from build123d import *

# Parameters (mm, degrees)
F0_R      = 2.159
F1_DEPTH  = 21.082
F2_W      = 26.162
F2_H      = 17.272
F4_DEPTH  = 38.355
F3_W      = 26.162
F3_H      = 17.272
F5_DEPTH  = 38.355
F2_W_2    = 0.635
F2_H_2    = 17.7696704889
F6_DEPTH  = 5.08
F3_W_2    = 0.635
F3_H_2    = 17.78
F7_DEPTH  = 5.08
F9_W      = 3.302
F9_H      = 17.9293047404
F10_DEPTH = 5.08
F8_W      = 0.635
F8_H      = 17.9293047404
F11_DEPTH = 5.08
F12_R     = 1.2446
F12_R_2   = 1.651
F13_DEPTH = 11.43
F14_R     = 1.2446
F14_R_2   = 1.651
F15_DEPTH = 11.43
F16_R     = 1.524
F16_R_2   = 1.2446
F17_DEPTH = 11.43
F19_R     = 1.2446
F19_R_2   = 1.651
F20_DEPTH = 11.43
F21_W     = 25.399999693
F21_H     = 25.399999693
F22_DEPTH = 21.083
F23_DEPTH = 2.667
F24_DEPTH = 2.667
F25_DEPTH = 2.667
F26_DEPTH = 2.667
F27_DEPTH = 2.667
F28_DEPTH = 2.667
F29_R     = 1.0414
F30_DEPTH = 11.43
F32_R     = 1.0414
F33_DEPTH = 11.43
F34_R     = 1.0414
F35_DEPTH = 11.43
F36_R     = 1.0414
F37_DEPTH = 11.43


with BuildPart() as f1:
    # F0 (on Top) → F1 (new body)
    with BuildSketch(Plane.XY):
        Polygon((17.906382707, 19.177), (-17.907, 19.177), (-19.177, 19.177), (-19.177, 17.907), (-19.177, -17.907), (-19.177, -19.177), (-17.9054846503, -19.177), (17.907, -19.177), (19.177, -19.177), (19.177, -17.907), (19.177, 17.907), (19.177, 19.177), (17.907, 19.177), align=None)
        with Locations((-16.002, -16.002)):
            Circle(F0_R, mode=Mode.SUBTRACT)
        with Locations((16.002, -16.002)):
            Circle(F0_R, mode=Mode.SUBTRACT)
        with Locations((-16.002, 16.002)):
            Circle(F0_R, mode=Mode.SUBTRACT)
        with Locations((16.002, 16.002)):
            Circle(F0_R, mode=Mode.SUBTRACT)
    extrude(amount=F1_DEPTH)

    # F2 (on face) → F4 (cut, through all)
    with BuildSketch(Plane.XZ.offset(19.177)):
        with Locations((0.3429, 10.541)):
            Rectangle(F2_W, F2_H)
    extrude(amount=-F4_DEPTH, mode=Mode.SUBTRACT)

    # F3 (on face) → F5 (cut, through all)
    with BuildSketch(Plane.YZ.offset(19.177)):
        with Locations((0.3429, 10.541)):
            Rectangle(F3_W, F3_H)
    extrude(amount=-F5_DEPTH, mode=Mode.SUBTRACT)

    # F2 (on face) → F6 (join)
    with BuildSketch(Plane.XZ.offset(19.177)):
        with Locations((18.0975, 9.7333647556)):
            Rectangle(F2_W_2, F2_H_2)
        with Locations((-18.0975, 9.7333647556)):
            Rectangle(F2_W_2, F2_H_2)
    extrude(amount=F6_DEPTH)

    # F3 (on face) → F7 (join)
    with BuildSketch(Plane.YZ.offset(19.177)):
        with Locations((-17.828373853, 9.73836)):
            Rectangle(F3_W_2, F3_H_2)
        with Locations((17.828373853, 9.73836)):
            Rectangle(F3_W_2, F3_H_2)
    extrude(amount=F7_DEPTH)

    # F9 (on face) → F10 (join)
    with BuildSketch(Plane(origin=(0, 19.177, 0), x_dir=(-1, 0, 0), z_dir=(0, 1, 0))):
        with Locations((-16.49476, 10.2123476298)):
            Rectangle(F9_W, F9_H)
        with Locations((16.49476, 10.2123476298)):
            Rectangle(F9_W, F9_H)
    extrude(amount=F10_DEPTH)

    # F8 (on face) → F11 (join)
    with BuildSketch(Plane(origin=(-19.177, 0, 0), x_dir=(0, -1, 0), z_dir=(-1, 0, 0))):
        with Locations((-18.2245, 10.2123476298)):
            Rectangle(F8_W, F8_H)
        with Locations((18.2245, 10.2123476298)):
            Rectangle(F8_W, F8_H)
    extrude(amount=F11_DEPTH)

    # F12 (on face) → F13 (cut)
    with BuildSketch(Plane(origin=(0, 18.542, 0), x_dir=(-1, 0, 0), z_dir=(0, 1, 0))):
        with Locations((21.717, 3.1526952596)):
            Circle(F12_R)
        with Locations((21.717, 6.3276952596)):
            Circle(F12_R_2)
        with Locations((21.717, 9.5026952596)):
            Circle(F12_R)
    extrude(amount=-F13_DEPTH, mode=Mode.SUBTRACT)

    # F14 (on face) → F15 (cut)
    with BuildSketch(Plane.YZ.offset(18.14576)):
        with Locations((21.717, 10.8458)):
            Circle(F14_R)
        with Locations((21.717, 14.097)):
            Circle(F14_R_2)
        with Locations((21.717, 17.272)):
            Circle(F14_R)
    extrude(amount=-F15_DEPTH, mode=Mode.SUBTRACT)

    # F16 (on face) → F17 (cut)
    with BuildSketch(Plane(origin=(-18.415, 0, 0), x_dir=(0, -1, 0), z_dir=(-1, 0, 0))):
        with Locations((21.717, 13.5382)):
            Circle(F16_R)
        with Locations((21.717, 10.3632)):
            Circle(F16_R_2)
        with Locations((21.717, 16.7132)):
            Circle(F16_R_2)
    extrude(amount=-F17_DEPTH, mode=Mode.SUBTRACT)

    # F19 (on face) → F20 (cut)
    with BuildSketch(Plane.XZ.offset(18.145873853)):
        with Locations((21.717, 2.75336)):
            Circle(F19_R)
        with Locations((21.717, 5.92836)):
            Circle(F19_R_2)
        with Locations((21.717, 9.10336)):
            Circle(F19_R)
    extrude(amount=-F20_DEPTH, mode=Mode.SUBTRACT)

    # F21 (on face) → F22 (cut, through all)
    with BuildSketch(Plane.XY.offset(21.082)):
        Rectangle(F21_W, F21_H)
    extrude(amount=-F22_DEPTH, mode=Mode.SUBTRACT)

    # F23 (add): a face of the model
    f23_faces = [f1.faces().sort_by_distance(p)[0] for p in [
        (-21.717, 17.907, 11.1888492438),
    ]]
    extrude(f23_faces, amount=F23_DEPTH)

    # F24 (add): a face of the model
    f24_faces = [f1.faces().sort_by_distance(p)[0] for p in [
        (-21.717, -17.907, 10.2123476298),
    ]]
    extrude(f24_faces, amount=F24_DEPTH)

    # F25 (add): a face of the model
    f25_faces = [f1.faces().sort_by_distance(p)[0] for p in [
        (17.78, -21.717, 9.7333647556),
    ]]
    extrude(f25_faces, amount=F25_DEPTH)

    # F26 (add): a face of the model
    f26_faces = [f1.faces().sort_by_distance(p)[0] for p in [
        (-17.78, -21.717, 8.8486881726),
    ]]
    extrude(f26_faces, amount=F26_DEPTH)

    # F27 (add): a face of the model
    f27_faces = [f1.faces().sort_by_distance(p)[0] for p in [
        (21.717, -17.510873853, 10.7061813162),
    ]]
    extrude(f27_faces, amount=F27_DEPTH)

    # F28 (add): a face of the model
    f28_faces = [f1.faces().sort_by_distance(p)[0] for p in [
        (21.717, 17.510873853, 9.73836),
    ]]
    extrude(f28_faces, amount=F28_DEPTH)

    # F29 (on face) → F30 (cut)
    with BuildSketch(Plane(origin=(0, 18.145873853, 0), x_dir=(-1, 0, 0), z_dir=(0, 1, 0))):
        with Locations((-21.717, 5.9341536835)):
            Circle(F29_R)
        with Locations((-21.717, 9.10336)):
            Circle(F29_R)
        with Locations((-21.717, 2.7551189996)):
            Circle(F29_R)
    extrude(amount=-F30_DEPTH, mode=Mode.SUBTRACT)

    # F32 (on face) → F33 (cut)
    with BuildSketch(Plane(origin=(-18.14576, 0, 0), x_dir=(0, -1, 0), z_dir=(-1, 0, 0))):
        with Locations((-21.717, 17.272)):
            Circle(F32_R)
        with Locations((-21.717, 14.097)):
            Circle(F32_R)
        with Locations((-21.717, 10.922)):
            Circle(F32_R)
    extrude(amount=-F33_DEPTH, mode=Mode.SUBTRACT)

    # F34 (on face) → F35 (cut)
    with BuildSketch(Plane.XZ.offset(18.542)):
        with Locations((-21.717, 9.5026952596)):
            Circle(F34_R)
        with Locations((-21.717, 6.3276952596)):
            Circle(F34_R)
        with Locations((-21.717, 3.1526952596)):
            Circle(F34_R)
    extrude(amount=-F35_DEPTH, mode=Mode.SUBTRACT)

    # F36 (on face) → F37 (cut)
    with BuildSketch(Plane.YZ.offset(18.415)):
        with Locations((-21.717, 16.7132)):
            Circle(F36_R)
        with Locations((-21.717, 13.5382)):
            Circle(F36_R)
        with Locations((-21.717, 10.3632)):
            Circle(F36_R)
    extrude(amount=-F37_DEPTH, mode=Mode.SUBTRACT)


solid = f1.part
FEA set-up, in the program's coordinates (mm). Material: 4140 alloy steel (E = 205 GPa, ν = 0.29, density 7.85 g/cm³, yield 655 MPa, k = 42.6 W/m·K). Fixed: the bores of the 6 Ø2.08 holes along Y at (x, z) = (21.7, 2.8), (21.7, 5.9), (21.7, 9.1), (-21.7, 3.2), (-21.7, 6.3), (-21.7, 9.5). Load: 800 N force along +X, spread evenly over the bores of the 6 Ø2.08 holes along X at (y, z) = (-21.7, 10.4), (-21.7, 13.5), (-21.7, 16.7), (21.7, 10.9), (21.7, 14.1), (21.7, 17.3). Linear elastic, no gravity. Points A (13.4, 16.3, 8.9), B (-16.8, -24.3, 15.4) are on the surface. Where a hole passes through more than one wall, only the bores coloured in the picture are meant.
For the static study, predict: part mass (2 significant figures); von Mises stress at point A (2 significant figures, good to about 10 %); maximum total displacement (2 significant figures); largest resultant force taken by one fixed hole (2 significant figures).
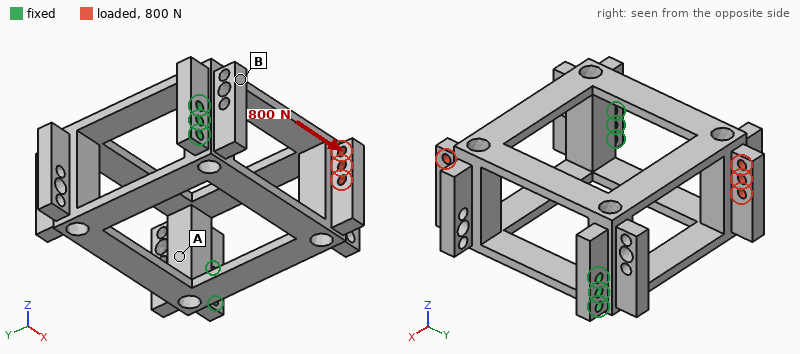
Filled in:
51 g
28 MPa
22 µm
550 N
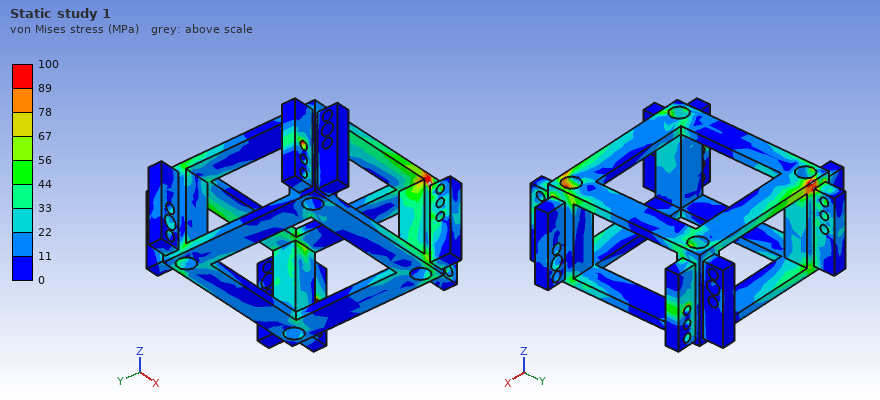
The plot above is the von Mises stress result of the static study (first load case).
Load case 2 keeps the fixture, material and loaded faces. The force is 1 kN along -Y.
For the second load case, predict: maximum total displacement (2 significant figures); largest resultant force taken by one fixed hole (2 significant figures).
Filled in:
27 µm
560 N
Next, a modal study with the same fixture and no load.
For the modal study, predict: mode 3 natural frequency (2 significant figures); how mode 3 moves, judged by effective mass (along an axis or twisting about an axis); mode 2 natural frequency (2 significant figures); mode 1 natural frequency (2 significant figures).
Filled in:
7500 Hz
along Y
1700 Hz
1700 Hz
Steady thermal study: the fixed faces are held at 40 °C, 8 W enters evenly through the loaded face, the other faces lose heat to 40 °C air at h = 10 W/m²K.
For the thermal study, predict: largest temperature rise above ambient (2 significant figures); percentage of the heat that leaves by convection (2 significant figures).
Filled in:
76 K
35 %
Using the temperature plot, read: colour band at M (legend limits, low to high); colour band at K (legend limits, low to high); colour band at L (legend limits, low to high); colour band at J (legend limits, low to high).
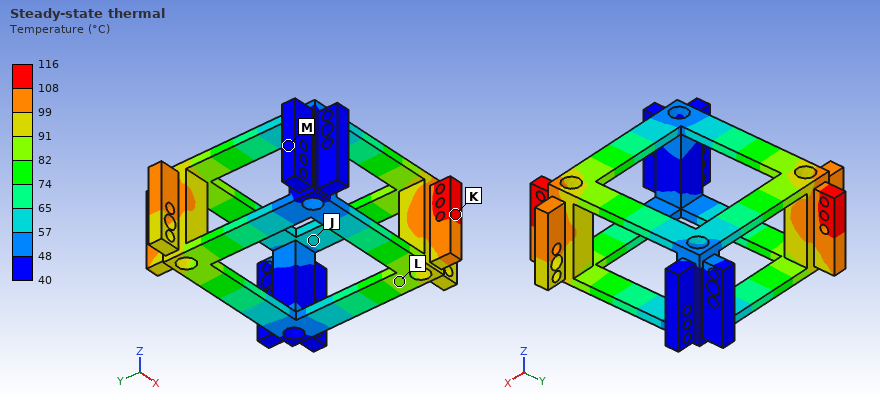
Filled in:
40 to 48 °C
108 to 116 °C
82 to 91 °C
57 to 65 °C
